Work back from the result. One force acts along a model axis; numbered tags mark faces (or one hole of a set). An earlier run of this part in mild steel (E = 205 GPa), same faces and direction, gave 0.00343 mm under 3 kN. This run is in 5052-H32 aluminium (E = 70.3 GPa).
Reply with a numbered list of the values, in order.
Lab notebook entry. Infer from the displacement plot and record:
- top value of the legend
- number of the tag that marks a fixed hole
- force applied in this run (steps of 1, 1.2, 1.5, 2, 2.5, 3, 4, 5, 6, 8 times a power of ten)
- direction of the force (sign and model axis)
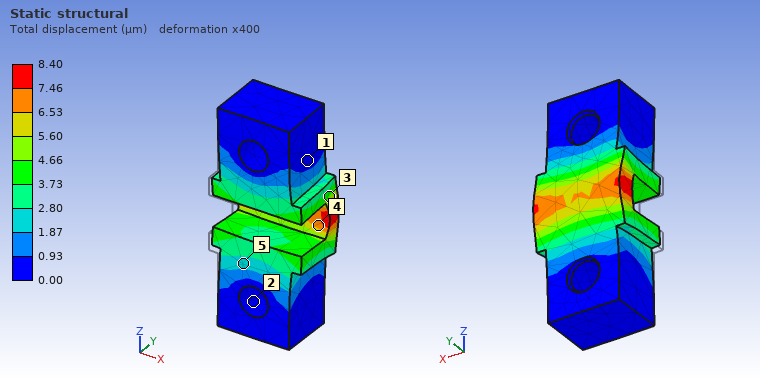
1. 8.40 µm
2. 2
3. 2.5 kN
4. +Y
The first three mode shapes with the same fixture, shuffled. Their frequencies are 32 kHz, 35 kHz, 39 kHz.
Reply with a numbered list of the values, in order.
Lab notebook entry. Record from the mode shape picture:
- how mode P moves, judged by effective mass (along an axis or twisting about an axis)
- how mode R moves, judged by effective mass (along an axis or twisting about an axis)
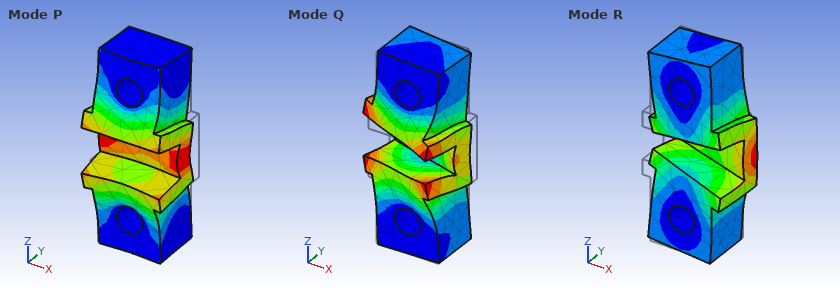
1. along Y
2. along X
